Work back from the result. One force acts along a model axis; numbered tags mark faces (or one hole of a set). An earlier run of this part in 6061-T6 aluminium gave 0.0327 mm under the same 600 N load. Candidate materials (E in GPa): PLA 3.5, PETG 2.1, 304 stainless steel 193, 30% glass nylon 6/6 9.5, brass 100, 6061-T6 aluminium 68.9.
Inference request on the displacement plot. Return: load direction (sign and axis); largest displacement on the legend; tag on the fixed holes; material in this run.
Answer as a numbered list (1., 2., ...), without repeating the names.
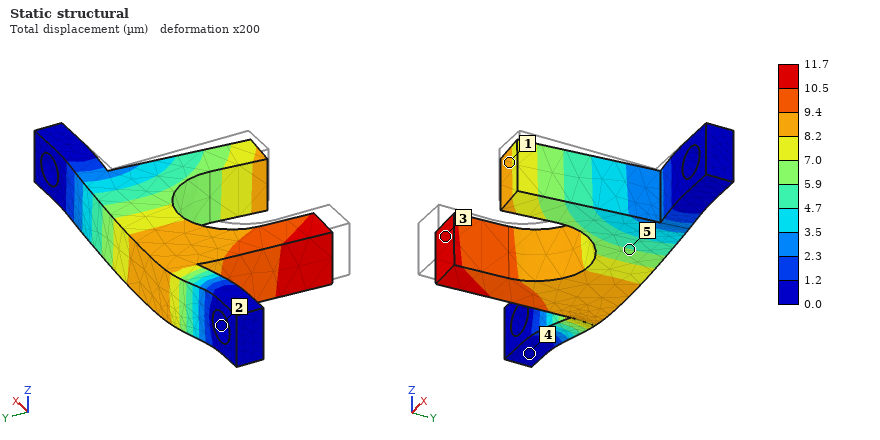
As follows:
1. +Y
2. 11.7 µm
3. 2
4. 304 stainless steel
